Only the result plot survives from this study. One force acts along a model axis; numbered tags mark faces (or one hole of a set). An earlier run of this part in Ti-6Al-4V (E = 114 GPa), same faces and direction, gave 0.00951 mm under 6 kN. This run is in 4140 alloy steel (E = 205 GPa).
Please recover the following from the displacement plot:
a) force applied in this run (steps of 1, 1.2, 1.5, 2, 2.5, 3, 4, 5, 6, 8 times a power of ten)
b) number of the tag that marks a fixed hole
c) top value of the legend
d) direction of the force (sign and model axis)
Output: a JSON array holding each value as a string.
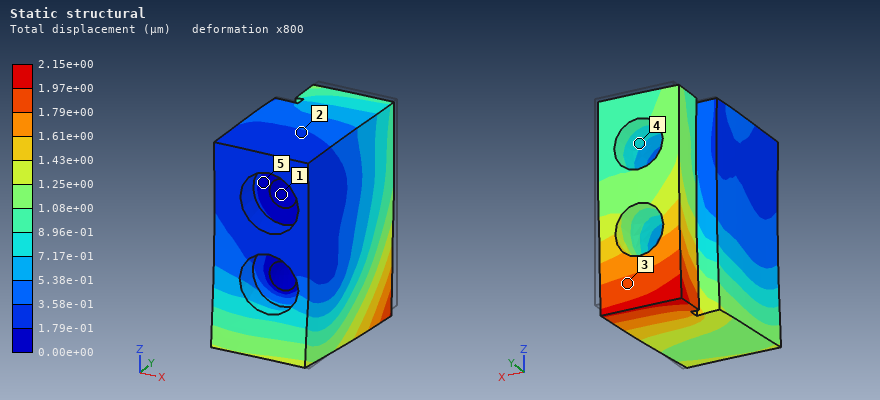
["2.5 kN", "1", "2.15e+00 µm", "-Y"]
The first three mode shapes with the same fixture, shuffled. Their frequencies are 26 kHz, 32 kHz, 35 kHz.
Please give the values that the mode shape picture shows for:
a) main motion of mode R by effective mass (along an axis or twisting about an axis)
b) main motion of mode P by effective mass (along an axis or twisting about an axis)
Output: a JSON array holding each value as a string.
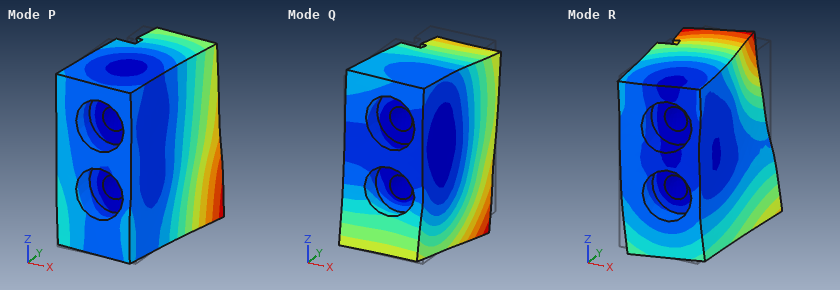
["twisting about Y", "along X"]
